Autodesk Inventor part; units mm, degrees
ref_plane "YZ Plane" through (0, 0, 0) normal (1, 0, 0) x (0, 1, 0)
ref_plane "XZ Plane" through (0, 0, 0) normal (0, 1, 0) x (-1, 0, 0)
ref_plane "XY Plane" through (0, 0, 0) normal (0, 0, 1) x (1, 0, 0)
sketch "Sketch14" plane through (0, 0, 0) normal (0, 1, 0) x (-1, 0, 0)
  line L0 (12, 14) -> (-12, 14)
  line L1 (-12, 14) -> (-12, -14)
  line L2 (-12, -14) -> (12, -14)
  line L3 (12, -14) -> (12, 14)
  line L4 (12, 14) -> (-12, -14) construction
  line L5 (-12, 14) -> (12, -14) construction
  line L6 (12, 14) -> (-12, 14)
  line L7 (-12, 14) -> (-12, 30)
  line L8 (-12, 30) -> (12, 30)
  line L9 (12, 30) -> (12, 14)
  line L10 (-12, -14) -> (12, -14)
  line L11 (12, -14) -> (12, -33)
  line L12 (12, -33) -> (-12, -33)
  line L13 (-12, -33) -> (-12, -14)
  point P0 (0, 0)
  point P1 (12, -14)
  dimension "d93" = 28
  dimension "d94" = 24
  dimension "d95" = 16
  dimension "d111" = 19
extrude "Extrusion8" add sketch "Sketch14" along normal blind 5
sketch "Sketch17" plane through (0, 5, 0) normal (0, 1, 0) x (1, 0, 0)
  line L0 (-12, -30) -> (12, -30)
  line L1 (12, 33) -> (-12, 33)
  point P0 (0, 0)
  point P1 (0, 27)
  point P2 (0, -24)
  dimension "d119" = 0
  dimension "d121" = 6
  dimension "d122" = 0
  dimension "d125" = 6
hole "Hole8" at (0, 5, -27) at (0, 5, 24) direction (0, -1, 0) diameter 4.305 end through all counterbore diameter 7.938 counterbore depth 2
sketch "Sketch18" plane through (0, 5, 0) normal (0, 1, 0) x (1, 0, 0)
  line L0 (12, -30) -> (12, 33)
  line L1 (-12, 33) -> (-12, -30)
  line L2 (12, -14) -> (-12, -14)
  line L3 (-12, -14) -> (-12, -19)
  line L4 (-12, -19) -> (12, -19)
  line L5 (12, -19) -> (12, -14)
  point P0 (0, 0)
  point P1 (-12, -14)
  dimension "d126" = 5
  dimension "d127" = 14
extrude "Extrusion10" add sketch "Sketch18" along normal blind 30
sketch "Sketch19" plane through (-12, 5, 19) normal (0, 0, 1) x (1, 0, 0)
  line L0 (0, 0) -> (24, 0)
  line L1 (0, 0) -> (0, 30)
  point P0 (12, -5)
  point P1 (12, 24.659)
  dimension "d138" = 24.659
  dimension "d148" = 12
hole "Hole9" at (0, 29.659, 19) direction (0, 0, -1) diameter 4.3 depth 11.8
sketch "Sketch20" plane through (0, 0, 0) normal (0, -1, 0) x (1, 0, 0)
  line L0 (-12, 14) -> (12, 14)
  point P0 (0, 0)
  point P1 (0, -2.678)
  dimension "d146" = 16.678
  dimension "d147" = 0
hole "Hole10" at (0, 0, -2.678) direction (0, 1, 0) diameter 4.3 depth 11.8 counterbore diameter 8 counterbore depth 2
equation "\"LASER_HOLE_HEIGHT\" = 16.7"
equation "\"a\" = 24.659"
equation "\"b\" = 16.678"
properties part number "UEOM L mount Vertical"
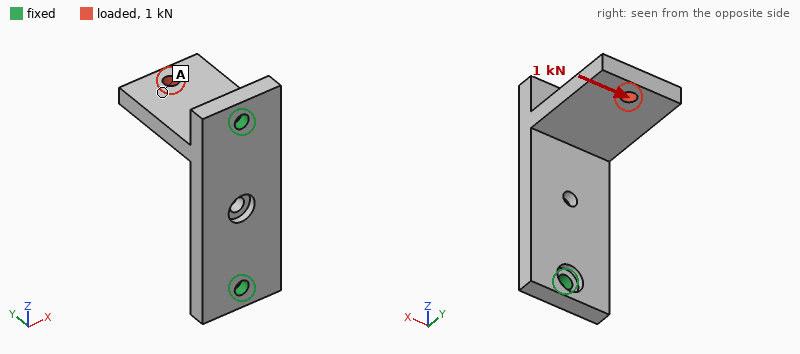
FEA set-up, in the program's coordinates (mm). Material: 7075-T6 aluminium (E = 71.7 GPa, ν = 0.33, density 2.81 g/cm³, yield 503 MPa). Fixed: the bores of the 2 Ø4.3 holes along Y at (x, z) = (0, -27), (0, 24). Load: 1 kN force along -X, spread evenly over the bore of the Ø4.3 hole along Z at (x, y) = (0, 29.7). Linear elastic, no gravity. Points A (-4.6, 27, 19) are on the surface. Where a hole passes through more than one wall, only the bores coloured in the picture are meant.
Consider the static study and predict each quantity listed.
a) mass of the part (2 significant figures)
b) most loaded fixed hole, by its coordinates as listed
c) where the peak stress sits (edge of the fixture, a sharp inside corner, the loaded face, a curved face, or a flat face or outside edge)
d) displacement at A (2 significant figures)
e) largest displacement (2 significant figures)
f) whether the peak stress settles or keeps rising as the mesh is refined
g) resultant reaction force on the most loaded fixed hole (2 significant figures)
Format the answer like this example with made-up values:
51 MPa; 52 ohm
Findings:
30 g; (0, 24); edge of the fixture; 0.32 mm; 0.43 mm; keeps rising; 850 N
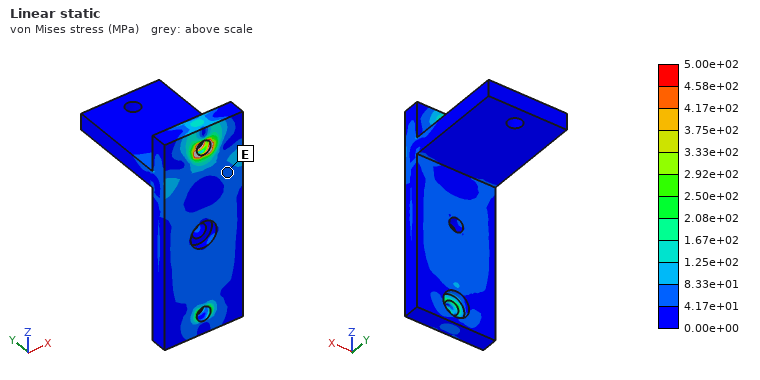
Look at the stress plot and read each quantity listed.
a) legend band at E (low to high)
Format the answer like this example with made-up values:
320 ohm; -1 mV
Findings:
4.17e+01 to 8.33e+01 MPa
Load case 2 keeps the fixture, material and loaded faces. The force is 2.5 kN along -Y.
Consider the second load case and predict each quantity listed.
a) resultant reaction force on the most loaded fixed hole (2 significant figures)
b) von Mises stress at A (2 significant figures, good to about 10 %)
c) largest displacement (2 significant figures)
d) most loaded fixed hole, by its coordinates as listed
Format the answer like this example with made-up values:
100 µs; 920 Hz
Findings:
2.4 kN; 33 MPa; 0.13 mm; (0, 24)
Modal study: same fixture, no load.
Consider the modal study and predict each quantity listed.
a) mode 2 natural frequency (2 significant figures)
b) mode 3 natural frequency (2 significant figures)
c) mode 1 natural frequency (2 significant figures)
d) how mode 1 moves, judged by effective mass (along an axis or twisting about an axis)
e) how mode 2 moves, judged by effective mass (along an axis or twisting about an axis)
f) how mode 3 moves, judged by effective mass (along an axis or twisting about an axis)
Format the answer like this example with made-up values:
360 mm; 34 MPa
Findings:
3400 Hz; 8200 Hz; 3100 Hz; along Z; along X; along Y
